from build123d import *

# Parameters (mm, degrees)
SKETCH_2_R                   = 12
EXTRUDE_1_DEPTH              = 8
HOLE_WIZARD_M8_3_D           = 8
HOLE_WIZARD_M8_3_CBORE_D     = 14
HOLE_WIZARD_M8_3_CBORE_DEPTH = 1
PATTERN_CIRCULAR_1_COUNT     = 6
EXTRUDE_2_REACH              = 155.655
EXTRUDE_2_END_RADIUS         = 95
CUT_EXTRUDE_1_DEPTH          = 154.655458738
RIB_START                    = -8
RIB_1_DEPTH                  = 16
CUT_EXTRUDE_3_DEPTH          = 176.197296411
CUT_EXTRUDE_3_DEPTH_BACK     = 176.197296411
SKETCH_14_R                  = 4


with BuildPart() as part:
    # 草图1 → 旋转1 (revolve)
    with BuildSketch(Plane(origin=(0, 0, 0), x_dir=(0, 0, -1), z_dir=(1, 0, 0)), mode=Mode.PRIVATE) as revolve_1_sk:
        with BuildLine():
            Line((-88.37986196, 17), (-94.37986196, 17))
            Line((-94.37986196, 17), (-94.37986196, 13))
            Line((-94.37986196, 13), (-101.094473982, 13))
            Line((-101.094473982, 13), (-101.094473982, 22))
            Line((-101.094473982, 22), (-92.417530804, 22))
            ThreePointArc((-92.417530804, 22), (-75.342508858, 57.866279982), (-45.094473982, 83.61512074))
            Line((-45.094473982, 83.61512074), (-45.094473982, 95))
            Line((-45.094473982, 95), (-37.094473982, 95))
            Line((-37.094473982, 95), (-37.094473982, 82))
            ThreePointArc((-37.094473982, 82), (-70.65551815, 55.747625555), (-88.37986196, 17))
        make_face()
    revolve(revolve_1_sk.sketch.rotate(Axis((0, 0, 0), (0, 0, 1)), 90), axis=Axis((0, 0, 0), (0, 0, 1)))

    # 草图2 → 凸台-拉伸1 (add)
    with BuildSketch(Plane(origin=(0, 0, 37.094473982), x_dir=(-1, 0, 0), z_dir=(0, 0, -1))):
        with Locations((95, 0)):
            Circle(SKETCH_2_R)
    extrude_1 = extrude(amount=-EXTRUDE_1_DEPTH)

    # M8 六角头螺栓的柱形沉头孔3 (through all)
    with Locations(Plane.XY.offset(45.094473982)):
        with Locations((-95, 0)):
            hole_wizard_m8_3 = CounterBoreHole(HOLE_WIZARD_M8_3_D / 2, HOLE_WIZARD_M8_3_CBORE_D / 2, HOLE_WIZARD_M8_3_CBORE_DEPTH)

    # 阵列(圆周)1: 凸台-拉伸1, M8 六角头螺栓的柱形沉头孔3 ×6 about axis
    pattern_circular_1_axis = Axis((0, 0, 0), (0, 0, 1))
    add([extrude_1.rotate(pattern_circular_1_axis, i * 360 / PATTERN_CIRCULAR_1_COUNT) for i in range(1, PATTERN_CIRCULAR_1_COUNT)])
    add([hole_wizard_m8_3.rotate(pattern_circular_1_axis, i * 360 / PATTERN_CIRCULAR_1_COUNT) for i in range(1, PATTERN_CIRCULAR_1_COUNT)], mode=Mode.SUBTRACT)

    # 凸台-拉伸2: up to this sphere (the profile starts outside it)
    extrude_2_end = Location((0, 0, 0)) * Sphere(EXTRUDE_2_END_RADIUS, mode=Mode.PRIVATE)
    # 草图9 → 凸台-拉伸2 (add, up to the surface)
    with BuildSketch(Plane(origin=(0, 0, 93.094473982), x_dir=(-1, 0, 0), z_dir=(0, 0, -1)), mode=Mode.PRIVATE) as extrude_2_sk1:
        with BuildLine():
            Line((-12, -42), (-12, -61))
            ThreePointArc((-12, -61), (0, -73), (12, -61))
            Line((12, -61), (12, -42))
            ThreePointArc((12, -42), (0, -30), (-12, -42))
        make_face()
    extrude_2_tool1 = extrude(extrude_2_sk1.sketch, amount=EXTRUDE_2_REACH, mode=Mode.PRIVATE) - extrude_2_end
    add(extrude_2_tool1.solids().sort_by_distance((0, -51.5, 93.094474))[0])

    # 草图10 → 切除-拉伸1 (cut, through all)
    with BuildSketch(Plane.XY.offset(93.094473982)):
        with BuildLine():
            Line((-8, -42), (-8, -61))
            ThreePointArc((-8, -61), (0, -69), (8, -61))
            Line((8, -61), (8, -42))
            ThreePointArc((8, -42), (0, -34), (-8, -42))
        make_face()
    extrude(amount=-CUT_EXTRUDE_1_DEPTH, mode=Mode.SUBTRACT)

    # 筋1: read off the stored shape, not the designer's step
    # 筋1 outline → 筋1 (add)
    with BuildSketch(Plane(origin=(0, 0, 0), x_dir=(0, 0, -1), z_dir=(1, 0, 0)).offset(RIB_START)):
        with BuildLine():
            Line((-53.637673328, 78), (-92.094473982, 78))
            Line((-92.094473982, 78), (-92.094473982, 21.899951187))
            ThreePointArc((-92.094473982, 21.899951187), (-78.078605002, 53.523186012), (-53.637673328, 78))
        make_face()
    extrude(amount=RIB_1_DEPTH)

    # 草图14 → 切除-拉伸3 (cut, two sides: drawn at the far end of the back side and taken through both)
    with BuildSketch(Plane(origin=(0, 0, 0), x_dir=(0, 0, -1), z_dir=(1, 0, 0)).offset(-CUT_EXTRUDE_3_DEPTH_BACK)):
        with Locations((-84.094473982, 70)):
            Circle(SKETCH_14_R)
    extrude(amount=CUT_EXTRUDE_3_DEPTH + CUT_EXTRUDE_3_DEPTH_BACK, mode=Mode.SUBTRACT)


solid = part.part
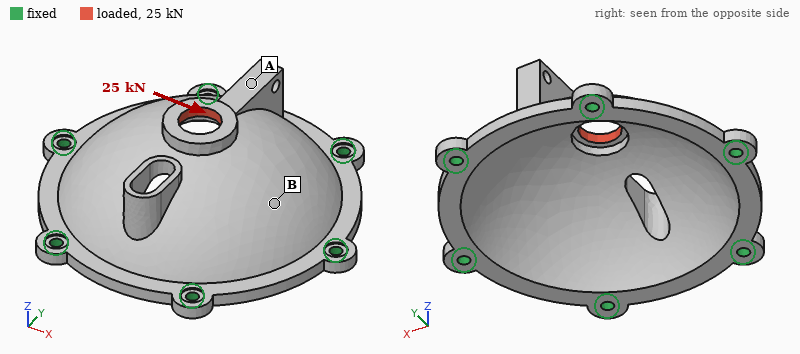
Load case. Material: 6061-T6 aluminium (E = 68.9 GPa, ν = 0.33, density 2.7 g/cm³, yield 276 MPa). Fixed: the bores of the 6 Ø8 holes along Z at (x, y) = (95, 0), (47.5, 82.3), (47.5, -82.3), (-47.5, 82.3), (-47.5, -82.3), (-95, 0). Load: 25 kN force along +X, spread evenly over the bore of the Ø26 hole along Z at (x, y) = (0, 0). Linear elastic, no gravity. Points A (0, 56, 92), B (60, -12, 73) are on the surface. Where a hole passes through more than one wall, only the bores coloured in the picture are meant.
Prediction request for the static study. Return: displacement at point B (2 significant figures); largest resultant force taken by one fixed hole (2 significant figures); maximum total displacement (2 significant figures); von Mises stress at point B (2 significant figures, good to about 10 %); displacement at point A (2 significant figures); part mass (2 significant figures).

0.061 mm
7.9 kN
0.13 mm
34 MPa
0.047 mm
620 g
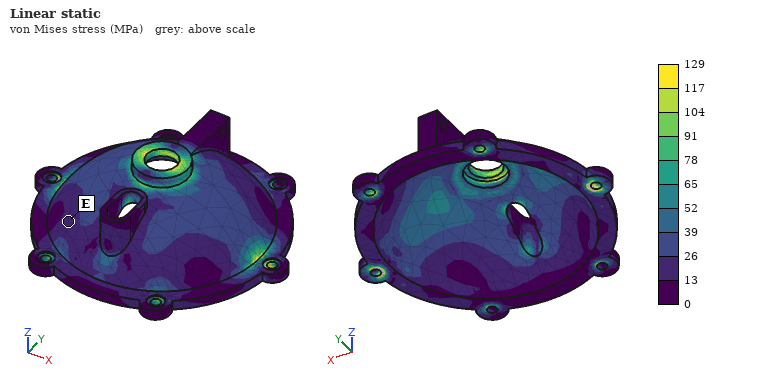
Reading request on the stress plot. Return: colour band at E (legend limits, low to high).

13 to 26 MPa
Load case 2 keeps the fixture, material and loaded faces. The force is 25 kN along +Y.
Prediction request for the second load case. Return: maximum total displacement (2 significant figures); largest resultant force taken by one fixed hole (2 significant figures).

0.13 mm
7.0 kN
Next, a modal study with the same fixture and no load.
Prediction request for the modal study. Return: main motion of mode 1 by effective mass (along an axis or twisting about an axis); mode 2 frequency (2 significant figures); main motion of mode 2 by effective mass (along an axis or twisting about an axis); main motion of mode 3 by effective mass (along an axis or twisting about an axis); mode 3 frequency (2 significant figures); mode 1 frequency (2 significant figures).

along Z
5200 Hz
along Z
along Z
5500 Hz
4900 Hz
